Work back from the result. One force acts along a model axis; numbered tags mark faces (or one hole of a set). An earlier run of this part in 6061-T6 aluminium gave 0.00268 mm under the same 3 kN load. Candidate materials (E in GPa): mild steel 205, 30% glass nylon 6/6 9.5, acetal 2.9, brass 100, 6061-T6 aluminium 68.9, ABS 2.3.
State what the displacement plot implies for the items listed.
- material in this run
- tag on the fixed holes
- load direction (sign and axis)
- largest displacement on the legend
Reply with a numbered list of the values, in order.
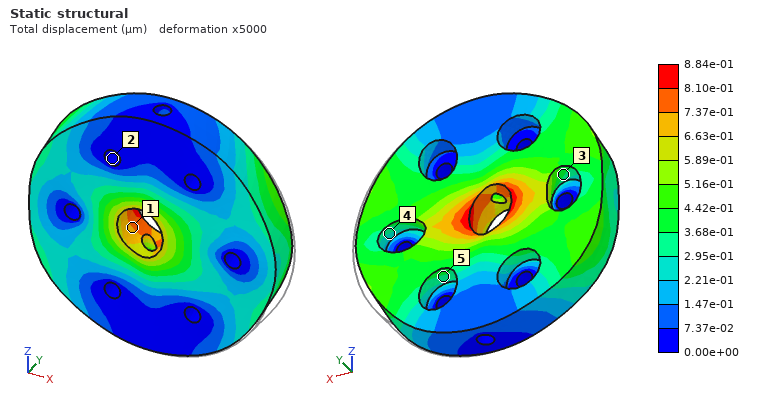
1. mild steel
2. 2
3. -X
4. 8.84e-01 µm
